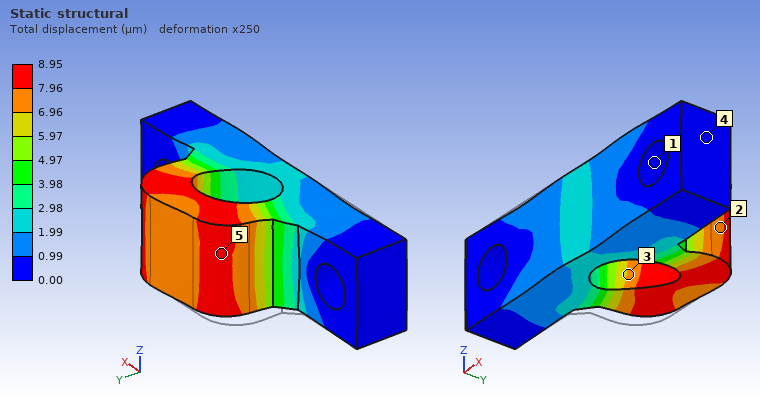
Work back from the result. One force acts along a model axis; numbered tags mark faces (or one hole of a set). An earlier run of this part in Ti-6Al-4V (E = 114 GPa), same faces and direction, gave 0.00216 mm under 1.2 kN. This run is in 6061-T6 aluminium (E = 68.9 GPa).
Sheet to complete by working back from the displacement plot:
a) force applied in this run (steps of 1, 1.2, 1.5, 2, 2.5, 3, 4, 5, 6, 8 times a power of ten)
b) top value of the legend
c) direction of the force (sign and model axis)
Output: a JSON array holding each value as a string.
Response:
["3 kN", "8.95 µm", "+X"]
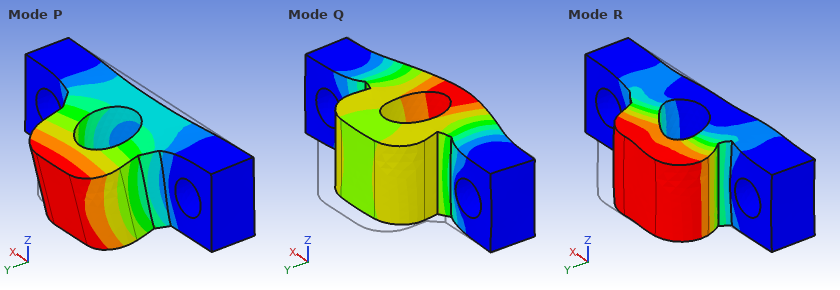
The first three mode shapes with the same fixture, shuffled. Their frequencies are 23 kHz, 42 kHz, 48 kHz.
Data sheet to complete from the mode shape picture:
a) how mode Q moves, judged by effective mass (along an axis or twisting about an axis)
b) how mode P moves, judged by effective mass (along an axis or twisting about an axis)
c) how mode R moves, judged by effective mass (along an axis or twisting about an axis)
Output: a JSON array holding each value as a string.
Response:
["along Y", "along Z", "along X"]
